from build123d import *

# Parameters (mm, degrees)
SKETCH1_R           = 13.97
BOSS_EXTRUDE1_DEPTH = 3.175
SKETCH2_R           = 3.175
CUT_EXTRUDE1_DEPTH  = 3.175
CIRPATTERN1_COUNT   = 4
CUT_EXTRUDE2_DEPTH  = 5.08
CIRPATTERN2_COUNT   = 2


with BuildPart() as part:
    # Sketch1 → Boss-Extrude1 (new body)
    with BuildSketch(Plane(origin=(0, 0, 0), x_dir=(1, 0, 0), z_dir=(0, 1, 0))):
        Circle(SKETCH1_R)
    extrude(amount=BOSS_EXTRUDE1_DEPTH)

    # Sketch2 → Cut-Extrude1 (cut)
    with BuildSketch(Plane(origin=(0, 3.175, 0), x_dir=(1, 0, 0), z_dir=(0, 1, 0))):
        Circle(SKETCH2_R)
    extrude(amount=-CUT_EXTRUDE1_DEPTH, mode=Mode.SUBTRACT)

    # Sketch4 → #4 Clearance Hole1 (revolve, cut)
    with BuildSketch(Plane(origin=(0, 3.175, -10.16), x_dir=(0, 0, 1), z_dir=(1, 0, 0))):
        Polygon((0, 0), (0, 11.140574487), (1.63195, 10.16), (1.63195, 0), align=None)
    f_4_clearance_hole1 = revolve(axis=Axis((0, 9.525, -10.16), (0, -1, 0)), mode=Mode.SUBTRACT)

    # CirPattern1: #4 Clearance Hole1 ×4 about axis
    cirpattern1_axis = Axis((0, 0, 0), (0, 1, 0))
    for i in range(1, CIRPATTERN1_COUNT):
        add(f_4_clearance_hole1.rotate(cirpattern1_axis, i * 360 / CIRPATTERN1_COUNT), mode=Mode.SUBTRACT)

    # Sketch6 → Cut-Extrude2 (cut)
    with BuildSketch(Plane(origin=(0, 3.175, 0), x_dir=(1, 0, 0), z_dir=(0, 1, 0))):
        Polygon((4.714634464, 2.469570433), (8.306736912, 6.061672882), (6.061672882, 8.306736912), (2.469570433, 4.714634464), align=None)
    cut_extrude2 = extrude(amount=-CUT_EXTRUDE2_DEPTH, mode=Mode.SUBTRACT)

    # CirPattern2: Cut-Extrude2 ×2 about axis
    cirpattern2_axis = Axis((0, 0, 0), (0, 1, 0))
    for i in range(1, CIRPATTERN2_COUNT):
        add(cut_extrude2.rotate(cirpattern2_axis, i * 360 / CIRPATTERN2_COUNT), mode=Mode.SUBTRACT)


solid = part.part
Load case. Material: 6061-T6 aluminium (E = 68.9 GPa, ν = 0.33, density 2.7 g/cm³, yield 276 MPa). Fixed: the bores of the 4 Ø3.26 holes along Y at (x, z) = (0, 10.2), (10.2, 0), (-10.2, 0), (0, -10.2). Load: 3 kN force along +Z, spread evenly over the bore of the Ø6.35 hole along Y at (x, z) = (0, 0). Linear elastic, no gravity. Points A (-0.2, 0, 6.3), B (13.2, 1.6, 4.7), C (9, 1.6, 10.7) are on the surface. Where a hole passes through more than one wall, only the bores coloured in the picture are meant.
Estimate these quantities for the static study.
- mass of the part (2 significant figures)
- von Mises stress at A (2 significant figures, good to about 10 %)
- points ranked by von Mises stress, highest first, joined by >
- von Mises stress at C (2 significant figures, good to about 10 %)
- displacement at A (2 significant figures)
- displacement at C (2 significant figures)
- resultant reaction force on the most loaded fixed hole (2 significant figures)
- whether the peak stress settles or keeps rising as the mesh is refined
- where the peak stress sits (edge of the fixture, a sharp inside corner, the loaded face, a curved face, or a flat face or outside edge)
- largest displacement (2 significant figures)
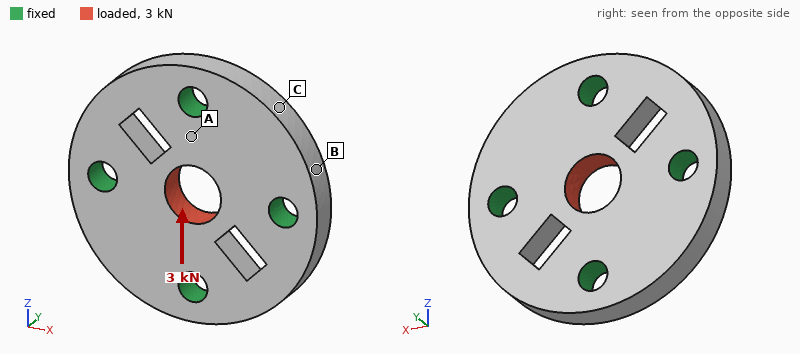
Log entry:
4.4 g
59 MPa
A > C > B
16 MPa
2.1 µm
2.0 µm
1.0 kN
keeps rising
a sharp inside corner
7.0 µm
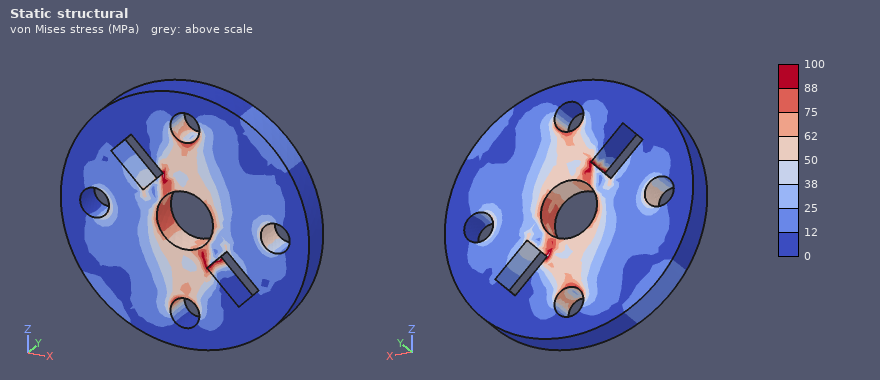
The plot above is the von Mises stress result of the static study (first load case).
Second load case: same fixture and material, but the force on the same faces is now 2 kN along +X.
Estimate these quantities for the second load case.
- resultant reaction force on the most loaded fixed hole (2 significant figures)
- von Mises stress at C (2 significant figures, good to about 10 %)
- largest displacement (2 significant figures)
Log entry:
670 N
9.8 MPa
4.6 µm
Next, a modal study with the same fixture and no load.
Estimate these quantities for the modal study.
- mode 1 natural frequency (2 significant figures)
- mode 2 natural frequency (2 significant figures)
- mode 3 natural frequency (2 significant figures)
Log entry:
51 kHz
53 kHz
53 kHz
